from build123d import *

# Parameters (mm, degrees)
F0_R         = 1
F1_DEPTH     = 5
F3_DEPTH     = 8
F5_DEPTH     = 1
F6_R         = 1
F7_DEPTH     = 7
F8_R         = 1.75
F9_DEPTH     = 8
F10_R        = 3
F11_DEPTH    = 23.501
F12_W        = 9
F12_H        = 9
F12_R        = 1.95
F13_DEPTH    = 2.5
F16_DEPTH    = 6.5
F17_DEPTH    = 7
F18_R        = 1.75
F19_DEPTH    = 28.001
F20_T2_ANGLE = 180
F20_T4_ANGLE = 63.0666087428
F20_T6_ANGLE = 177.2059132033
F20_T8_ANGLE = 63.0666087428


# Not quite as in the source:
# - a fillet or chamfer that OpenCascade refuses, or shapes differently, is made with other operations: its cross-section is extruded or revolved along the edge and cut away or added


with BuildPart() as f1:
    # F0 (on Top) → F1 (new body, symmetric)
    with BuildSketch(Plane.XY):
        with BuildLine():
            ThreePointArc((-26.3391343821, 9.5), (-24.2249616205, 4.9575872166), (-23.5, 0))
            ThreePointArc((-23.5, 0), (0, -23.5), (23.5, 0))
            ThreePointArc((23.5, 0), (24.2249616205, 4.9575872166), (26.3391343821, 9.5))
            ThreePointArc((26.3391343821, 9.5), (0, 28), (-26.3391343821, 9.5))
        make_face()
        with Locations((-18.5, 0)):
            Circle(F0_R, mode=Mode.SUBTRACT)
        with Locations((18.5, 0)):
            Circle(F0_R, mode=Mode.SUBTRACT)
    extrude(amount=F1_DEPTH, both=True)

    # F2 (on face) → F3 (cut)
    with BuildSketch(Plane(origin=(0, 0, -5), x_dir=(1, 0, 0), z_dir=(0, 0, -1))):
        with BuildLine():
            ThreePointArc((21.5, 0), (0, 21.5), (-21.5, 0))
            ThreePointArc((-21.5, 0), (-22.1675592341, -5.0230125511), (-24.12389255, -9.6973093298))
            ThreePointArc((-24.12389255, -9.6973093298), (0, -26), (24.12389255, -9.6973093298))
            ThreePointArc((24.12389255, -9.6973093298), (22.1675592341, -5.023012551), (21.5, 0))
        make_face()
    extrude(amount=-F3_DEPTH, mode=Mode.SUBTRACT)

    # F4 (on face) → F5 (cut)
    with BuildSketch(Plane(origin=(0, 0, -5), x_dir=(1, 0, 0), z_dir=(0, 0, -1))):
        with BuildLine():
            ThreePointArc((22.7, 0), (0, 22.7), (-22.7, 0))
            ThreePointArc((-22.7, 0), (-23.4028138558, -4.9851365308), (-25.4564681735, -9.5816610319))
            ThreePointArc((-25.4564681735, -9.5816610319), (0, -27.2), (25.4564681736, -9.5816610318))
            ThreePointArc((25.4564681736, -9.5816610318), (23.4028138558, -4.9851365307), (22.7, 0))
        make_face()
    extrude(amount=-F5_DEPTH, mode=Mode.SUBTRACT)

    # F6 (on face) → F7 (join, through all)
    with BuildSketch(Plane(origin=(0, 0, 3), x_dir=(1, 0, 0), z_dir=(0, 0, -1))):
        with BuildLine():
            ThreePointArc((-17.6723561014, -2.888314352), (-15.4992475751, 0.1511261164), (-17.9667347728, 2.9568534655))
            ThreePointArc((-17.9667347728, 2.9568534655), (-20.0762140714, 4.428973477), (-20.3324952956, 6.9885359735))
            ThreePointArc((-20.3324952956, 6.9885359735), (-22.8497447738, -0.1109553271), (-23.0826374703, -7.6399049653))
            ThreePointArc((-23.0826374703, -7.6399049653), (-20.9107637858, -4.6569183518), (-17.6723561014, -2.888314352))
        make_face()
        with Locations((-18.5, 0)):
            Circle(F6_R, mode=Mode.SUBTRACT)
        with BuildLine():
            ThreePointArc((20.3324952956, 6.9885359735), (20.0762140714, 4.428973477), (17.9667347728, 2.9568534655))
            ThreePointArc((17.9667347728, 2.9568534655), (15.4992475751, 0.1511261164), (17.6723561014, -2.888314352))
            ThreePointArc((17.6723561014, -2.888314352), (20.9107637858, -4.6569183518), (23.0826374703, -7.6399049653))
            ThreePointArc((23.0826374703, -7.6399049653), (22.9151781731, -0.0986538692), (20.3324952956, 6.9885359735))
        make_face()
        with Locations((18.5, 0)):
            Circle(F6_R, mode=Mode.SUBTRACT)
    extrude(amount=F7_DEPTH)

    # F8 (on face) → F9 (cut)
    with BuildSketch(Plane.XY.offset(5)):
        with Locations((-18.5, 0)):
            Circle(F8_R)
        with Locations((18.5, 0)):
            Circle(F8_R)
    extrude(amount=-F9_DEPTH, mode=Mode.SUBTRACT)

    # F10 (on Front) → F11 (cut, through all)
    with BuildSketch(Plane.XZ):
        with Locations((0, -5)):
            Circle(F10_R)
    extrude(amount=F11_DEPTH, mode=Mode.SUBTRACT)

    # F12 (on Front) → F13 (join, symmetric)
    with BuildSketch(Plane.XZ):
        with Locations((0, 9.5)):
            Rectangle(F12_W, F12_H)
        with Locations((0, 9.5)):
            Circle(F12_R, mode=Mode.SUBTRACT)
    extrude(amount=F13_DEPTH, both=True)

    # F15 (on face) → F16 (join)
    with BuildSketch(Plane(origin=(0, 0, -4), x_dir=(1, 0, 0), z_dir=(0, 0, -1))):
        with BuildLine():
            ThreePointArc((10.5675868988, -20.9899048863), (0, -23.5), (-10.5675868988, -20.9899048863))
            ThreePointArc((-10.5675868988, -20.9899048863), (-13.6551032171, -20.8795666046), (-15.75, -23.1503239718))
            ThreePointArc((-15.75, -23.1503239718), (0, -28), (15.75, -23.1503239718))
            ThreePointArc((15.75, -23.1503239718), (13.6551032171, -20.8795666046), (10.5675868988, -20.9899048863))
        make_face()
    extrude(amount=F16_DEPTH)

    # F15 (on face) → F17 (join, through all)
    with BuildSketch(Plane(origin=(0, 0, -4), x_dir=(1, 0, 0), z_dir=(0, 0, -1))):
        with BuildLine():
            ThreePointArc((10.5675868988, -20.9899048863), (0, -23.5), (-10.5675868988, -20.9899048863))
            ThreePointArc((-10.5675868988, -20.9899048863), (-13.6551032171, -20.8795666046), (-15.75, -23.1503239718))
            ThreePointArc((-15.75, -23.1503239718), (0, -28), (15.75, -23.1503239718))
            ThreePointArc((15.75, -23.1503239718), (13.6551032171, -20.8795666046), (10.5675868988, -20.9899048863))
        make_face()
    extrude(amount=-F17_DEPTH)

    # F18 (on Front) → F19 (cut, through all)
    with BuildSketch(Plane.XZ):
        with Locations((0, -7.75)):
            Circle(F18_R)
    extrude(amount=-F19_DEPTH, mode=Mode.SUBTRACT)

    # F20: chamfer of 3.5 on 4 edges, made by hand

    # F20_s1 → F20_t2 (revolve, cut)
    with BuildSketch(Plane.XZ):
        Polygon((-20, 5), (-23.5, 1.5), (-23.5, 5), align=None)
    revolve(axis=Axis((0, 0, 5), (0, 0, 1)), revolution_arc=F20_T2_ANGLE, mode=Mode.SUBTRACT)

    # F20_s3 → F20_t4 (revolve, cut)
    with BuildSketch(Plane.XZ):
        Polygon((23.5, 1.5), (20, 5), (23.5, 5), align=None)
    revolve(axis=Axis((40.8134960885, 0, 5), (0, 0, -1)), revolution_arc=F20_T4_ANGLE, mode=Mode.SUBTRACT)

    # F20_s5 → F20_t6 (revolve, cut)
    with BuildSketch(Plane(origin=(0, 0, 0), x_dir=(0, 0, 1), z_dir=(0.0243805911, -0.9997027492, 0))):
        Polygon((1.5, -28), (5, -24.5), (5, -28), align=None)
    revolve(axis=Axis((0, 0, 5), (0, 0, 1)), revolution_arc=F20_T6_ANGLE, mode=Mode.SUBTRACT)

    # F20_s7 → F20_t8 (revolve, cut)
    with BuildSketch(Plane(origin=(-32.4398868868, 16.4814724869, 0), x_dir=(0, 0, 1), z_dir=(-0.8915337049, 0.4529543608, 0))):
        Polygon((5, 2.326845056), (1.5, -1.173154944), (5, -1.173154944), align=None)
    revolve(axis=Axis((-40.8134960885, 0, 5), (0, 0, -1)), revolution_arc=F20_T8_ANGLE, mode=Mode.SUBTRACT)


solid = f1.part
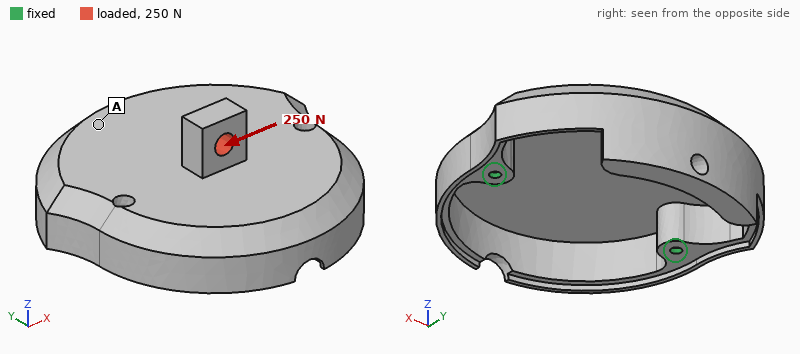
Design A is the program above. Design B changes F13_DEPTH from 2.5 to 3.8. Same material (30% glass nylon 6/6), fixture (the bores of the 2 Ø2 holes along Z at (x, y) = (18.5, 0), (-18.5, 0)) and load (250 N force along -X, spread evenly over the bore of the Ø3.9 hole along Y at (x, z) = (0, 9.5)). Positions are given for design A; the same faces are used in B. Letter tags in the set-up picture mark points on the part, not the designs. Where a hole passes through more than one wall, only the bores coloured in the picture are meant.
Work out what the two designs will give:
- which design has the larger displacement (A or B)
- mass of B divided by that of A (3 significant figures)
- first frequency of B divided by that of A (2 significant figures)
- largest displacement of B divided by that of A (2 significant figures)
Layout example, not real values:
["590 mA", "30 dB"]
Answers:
["A", "1.02", "0.99", "0.89"]
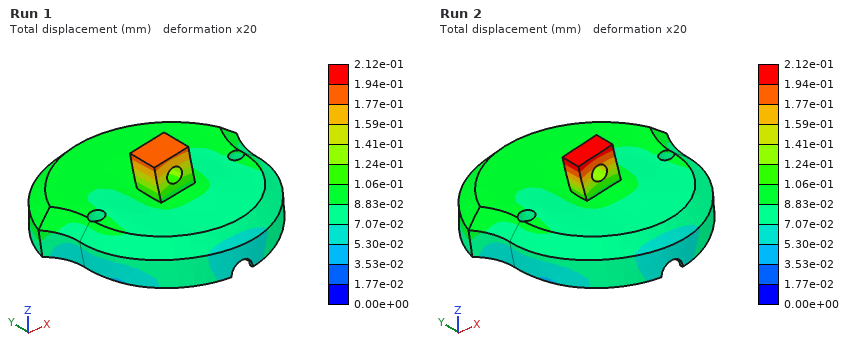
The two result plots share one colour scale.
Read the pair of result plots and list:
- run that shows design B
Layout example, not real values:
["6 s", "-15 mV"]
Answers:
["Run 1"]
